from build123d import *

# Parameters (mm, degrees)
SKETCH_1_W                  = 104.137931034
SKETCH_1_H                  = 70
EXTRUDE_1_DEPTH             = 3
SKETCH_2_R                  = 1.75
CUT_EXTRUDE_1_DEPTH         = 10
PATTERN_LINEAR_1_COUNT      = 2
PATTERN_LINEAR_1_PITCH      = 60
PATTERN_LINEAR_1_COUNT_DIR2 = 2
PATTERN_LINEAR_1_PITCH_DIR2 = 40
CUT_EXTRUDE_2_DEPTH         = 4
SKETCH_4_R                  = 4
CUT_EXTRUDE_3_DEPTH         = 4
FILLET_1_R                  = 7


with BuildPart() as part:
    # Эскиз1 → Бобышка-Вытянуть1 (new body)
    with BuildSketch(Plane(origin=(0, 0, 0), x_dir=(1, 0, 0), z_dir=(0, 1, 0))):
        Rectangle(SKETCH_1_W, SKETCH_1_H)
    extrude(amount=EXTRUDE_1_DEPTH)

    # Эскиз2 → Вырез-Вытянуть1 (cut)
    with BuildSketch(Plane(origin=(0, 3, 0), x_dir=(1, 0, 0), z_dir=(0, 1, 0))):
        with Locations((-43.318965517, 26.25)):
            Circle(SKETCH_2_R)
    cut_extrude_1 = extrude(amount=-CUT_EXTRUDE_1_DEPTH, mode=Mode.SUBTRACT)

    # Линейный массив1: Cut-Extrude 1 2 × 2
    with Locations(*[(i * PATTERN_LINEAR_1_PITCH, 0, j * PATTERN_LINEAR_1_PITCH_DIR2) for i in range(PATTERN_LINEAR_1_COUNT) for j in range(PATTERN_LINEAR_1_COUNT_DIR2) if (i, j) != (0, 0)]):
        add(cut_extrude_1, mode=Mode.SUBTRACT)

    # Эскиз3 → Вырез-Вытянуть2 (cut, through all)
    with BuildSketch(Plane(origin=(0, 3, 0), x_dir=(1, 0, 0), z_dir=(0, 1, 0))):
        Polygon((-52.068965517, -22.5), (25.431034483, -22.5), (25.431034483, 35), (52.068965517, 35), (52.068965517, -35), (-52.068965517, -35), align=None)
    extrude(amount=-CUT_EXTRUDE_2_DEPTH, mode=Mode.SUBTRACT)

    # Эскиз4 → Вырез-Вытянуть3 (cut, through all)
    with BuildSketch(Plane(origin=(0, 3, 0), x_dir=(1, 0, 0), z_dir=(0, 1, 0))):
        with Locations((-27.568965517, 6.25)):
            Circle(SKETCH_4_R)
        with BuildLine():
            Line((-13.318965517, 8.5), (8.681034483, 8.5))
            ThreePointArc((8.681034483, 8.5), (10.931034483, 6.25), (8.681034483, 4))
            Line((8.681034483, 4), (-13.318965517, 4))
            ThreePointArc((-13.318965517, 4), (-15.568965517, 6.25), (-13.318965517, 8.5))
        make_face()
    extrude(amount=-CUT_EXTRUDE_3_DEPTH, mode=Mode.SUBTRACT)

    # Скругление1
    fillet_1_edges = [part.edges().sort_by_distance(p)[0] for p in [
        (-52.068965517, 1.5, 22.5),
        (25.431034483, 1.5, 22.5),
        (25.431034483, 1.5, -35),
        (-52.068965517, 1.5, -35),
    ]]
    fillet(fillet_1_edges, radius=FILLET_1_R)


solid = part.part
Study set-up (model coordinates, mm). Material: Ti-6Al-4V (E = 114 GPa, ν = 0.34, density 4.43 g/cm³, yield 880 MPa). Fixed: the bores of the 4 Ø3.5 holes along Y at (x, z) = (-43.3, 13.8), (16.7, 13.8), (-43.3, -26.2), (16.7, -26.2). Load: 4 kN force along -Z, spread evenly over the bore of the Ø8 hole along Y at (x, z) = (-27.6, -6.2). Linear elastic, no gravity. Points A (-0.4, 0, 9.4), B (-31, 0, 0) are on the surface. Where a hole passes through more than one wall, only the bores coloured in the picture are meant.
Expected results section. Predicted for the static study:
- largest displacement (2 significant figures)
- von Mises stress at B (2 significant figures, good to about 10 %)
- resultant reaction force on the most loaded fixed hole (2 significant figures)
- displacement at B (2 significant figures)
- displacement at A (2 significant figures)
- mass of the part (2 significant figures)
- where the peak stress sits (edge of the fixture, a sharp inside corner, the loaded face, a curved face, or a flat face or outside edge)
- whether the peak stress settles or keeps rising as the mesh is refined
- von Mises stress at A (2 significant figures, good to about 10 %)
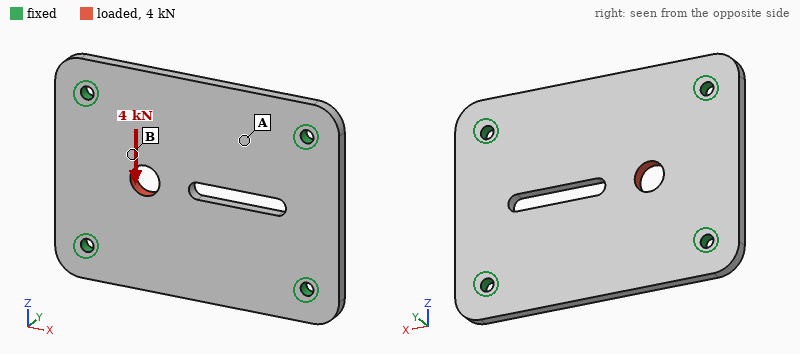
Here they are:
12 µm
47 MPa
1.7 kN
8.7 µm
4.6 µm
56 g
edge of the fixture
keeps rising
15 MPa
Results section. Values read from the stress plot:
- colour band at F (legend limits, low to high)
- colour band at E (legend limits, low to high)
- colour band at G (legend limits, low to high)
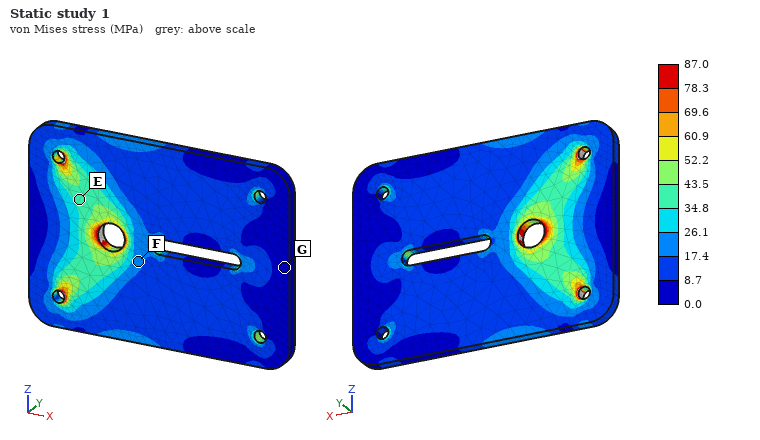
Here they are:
17.4 to 26.1 MPa
34.8 to 43.5 MPa
0.0 to 8.7 MPa
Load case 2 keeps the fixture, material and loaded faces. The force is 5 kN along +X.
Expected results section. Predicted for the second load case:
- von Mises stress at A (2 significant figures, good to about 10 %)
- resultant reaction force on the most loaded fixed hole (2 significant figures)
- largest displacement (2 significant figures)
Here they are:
18 MPa
1.6 kN
13 µm
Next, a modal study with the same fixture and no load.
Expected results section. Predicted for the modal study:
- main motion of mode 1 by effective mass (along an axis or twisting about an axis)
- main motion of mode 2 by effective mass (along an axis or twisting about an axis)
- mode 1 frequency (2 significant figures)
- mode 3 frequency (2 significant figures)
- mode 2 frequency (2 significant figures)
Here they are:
along Y
twisting about X
3800 Hz
6700 Hz
5000 Hz
